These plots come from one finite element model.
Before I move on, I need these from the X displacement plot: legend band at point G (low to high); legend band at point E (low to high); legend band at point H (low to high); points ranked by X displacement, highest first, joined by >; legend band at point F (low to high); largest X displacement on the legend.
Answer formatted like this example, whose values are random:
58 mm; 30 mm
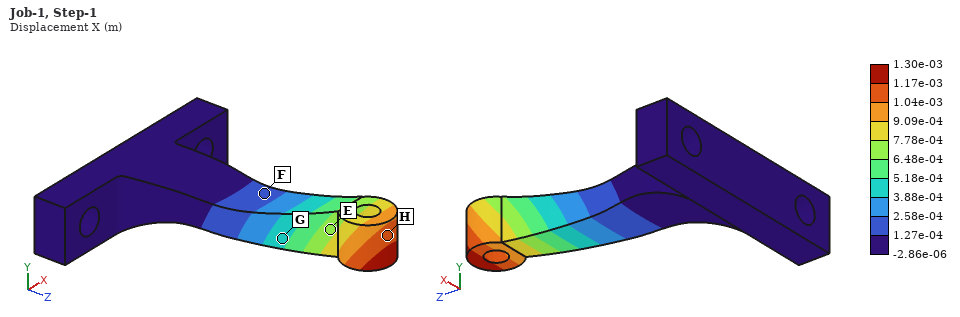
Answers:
3.88e-04 to 5.18e-04 m; 6.48e-04 to 7.78e-04 m; 1.04e-03 to 1.17e-03 m; H > E > G > F; 1.27e-04 to 2.58e-04 m; 1.30e-03 m
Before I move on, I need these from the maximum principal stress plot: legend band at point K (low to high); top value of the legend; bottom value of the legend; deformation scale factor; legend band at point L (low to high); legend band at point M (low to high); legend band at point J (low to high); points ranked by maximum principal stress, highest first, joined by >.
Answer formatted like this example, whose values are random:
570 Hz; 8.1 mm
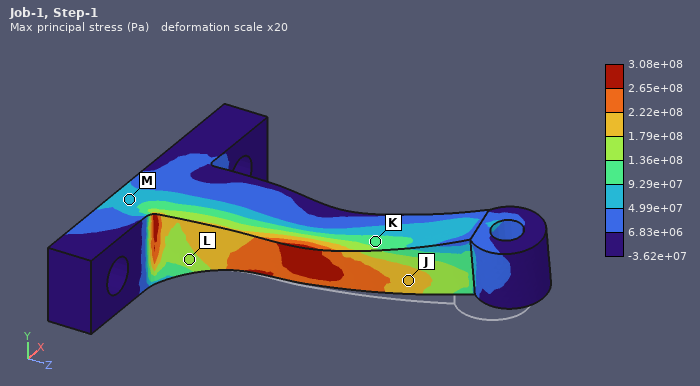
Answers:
9.29e+07 to 1.36e+08 Pa; 3.08e+08 Pa; -3.62e+07 Pa; 20; 1.36e+08 to 1.79e+08 Pa; 4.99e+07 to 9.29e+07 Pa; 1.79e+08 to 2.22e+08 Pa; J > L > K > M
